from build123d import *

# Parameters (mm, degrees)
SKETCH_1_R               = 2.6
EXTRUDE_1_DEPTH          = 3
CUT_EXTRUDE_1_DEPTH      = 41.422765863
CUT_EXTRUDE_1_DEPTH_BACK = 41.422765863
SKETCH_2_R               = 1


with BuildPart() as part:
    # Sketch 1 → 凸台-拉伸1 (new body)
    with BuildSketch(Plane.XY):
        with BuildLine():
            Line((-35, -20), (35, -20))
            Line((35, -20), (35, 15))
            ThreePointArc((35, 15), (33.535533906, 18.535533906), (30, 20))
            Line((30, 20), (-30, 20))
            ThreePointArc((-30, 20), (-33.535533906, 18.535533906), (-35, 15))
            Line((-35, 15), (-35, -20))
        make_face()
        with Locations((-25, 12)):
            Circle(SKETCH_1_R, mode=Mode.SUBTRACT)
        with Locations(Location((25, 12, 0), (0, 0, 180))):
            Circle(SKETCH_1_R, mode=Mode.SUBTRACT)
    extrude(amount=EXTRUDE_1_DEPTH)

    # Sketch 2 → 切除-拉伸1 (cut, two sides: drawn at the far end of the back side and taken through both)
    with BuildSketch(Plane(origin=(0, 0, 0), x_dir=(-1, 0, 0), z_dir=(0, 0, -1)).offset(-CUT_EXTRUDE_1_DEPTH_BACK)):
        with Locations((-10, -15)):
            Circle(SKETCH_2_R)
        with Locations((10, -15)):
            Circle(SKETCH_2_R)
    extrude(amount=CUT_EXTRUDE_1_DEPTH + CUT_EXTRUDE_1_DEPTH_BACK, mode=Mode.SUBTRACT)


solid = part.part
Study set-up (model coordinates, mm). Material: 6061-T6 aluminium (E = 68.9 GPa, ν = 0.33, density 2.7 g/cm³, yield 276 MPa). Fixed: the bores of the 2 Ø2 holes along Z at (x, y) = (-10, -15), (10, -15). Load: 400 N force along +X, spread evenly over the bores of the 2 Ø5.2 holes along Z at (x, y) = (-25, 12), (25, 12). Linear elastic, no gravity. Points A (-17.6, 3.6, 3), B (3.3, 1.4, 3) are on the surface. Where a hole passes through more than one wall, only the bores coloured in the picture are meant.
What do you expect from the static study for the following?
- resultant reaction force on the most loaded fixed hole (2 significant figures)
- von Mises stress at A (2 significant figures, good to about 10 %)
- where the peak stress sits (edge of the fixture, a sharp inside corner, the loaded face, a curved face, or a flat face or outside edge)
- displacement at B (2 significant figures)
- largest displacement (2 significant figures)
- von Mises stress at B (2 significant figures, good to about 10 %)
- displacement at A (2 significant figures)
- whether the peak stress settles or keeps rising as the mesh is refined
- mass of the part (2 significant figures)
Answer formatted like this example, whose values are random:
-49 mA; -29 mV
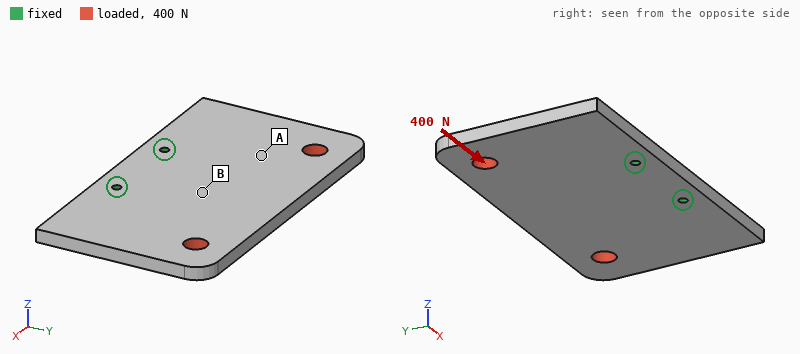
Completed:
550 N; 4.2 MPa; edge of the fixture; 7.0 µm; 19 µm; 9.3 MPa; 10.0 µm; keeps rising; 22 g
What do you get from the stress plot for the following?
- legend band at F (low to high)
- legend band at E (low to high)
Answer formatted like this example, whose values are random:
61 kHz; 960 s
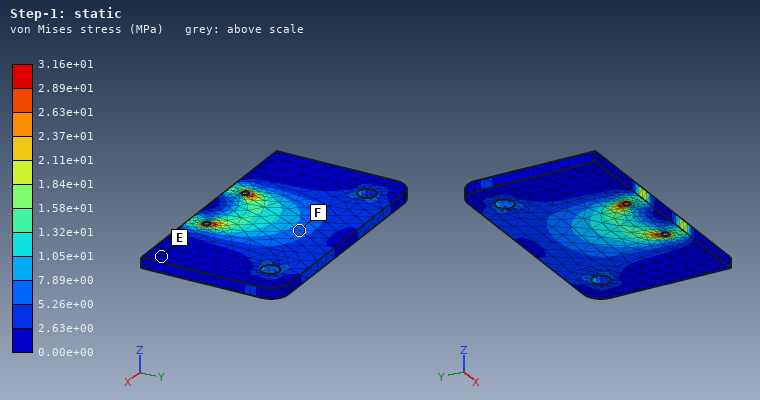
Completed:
5.26e+00 to 7.89e+00 MPa; 0.00e+00 to 2.63e+00 MPa
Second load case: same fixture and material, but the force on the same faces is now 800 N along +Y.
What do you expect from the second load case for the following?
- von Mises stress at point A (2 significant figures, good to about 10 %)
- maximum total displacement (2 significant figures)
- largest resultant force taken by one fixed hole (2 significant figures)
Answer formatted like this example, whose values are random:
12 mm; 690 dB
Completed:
8.5 MPa; 6.7 µm; 420 N
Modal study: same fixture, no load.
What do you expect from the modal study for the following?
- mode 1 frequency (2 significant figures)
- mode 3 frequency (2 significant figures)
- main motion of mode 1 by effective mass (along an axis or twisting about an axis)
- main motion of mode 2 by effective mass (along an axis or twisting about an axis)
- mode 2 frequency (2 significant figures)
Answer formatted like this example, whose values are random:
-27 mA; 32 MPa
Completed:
1500 Hz; 3400 Hz; along Z; twisting about Y; 1900 Hz
